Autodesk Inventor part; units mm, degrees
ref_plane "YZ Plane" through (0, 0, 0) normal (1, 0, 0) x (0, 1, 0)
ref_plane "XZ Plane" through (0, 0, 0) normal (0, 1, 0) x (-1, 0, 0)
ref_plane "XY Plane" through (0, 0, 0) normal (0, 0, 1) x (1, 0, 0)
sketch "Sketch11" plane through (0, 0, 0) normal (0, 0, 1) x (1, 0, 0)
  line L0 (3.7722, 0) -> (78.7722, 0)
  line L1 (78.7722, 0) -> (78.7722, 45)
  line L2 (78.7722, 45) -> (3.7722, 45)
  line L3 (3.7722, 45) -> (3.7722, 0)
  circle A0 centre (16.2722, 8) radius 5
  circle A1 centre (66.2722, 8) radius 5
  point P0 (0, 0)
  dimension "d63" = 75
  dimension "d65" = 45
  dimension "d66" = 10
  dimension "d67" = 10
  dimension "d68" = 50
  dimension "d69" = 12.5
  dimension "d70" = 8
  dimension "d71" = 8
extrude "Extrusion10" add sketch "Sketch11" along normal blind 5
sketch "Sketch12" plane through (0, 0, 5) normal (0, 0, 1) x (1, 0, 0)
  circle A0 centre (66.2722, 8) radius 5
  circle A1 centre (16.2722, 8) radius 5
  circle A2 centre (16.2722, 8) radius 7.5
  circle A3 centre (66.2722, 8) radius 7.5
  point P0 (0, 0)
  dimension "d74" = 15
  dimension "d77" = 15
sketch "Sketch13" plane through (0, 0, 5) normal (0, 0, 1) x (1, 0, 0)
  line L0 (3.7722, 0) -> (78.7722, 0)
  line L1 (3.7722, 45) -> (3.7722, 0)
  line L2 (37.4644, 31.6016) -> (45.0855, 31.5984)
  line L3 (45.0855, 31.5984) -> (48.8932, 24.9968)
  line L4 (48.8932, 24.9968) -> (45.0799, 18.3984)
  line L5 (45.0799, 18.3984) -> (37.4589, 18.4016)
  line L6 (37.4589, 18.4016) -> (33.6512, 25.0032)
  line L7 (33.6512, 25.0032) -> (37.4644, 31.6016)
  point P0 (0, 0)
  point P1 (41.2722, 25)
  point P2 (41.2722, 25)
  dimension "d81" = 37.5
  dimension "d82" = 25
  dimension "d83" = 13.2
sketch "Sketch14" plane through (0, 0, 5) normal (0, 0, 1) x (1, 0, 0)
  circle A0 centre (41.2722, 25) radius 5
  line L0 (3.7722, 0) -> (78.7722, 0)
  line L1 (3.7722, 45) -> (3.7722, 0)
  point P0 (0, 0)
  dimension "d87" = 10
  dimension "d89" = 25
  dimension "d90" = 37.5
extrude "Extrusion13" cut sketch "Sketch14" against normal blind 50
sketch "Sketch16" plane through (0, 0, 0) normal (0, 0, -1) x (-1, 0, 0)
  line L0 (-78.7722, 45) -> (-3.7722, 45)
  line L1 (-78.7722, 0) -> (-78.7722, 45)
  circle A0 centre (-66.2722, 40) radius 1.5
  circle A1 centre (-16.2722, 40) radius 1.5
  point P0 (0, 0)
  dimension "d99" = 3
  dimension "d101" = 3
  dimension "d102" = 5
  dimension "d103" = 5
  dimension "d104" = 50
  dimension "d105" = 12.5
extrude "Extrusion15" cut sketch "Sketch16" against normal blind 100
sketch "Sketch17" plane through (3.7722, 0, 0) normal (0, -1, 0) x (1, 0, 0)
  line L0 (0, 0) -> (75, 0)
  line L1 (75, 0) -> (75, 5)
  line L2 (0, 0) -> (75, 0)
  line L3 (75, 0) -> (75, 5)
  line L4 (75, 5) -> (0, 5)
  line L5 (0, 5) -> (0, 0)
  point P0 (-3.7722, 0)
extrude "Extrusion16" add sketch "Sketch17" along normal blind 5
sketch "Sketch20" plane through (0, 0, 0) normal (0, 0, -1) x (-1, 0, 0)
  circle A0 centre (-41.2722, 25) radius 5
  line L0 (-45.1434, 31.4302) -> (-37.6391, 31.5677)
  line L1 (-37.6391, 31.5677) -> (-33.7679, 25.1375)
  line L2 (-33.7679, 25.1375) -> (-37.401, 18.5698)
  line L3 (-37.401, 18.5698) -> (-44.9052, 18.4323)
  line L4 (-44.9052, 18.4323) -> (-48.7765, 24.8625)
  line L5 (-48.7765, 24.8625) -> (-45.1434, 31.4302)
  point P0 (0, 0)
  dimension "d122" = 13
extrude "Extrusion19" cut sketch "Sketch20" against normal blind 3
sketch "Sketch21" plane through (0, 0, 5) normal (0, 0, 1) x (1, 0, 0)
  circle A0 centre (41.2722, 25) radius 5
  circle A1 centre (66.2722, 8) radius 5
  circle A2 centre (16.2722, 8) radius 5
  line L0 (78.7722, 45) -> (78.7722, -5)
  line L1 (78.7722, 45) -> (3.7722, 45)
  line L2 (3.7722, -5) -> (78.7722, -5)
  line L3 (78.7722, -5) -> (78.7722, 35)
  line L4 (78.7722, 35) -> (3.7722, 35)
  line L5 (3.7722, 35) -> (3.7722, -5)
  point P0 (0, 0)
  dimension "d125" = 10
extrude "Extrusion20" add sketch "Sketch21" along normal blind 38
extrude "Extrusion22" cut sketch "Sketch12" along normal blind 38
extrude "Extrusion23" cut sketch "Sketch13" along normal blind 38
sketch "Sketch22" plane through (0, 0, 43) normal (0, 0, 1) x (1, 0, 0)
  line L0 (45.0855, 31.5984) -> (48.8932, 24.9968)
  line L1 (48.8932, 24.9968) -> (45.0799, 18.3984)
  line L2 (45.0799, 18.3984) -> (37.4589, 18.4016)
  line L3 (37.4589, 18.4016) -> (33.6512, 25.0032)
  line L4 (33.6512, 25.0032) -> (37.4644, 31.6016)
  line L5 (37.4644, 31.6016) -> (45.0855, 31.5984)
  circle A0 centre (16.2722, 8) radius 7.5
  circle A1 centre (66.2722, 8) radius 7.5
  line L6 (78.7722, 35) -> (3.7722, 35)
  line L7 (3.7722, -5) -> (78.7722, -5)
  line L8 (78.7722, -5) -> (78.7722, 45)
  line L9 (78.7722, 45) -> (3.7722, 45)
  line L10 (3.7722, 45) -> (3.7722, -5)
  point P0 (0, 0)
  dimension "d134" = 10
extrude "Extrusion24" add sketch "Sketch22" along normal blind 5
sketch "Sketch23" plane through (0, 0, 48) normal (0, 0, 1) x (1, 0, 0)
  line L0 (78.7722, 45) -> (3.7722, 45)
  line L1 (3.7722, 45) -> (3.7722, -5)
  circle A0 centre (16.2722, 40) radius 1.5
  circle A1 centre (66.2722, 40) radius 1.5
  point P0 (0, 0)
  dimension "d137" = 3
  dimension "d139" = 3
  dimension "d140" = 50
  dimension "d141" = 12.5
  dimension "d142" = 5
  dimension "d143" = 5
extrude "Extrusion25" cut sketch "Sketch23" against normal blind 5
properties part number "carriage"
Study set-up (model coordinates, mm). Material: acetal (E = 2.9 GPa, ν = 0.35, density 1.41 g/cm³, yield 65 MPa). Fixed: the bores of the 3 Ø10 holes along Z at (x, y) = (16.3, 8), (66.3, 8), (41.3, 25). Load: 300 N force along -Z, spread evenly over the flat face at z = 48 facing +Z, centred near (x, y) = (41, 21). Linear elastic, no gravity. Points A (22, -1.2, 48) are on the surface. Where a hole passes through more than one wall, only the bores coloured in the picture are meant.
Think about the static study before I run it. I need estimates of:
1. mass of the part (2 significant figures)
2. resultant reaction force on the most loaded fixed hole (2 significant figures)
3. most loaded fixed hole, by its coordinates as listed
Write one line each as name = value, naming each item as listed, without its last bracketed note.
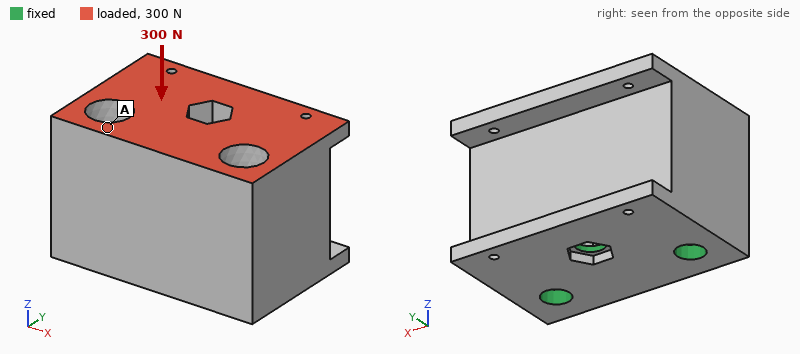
mass of the part = 180 g
resultant reaction force on the most loaded fixed hole = 170 N
most loaded fixed hole, by its coordinates as listed = (41.3, 25)
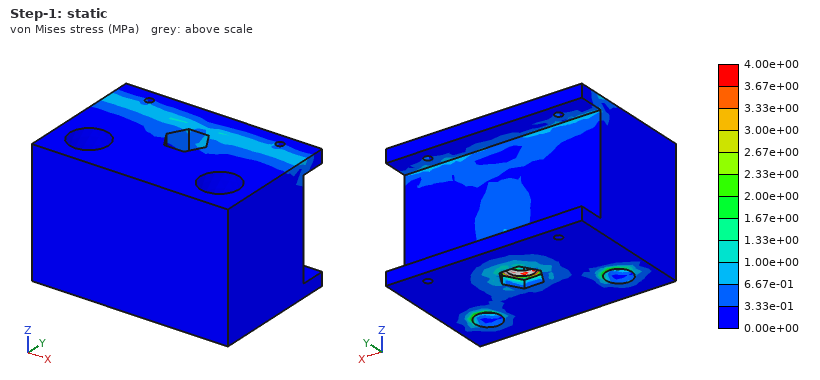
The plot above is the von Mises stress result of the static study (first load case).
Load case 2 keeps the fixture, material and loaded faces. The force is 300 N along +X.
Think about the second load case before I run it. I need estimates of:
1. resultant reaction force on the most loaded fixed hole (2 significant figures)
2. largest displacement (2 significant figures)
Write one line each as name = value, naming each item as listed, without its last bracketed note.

resultant reaction force on the most loaded fixed hole = 280 N
largest displacement = 37 µm
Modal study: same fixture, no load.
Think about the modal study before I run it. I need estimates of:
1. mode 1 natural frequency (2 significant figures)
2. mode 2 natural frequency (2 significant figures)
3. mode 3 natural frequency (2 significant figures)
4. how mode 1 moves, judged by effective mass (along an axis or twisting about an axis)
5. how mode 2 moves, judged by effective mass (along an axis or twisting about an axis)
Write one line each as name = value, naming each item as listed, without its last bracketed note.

mode 1 natural frequency = 950 Hz
mode 2 natural frequency = 1900 Hz
mode 3 natural frequency = 2500 Hz
how mode 1 moves, judged by effective mass = along Y
how mode 2 moves, judged by effective mass = along X
